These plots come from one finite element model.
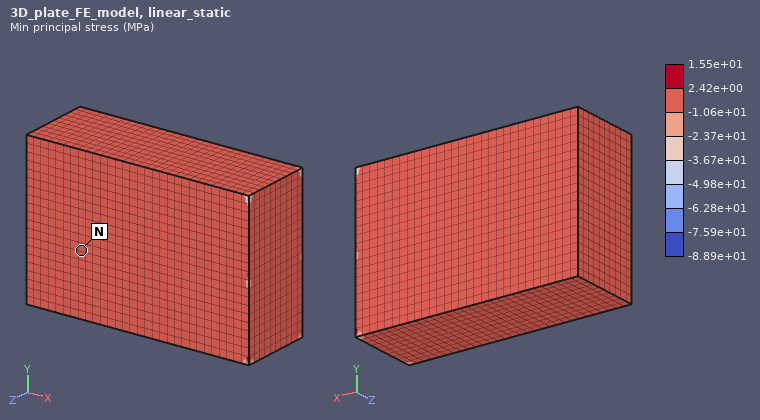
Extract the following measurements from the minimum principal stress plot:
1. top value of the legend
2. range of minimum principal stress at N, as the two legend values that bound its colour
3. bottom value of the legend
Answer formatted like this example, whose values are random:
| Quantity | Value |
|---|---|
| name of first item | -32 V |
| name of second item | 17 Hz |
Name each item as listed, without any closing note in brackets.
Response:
| Quantity | Value |
|---|---|
| top value of the legend | 1.55e+01 MPa |
| range of minimum principal stress at N, as the two legend values that bound its colour | -1.06e+01 to 2.42e+00 MPa |
| bottom value of the legend | -8.89e+01 MPa |
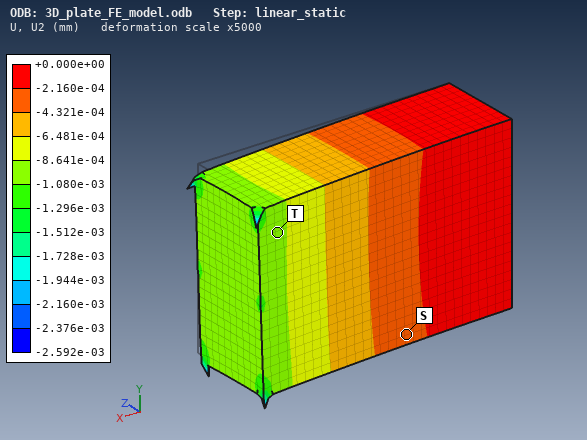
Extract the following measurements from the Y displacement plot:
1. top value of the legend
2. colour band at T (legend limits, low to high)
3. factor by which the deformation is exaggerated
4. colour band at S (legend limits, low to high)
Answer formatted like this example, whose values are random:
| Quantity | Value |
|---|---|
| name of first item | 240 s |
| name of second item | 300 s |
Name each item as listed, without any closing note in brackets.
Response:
| Quantity | Value |
|---|---|
| top value of the legend | +0.000e+00 mm |
| colour band at T | -1.080e-03 to -8.641e-04 mm |
| factor by which the deformation is exaggerated | 5000 |
| colour band at S | -4.321e-04 to -2.160e-04 mm |
